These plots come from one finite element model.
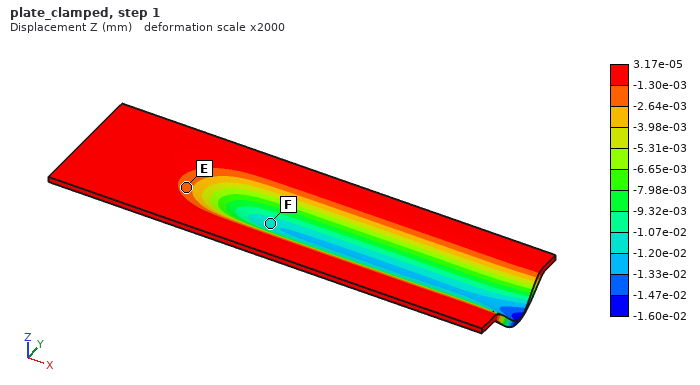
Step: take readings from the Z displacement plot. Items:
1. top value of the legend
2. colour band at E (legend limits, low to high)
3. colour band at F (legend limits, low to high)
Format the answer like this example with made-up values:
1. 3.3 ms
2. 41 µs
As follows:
1. 3.17e-05 mm
2. -2.64e-03 to -1.30e-03 mm
3. -1.20e-02 to -1.07e-02 mm
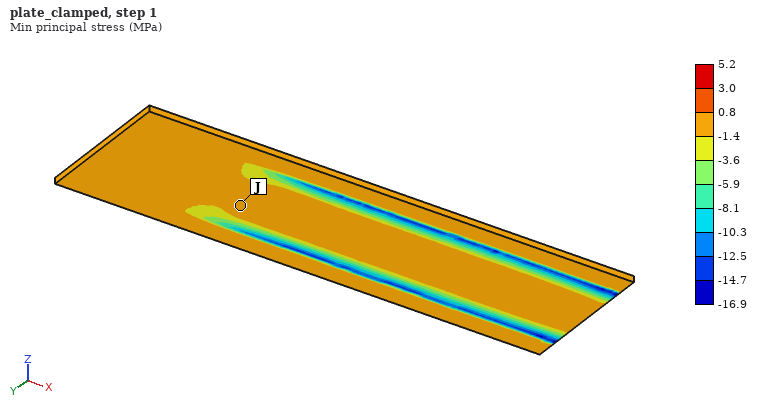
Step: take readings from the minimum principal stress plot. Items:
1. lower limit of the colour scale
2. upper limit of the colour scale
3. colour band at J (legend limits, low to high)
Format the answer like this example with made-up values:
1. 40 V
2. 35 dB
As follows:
1. -16.9 MPa
2. 5.2 MPa
3. -1.4 to 0.8 MPa
